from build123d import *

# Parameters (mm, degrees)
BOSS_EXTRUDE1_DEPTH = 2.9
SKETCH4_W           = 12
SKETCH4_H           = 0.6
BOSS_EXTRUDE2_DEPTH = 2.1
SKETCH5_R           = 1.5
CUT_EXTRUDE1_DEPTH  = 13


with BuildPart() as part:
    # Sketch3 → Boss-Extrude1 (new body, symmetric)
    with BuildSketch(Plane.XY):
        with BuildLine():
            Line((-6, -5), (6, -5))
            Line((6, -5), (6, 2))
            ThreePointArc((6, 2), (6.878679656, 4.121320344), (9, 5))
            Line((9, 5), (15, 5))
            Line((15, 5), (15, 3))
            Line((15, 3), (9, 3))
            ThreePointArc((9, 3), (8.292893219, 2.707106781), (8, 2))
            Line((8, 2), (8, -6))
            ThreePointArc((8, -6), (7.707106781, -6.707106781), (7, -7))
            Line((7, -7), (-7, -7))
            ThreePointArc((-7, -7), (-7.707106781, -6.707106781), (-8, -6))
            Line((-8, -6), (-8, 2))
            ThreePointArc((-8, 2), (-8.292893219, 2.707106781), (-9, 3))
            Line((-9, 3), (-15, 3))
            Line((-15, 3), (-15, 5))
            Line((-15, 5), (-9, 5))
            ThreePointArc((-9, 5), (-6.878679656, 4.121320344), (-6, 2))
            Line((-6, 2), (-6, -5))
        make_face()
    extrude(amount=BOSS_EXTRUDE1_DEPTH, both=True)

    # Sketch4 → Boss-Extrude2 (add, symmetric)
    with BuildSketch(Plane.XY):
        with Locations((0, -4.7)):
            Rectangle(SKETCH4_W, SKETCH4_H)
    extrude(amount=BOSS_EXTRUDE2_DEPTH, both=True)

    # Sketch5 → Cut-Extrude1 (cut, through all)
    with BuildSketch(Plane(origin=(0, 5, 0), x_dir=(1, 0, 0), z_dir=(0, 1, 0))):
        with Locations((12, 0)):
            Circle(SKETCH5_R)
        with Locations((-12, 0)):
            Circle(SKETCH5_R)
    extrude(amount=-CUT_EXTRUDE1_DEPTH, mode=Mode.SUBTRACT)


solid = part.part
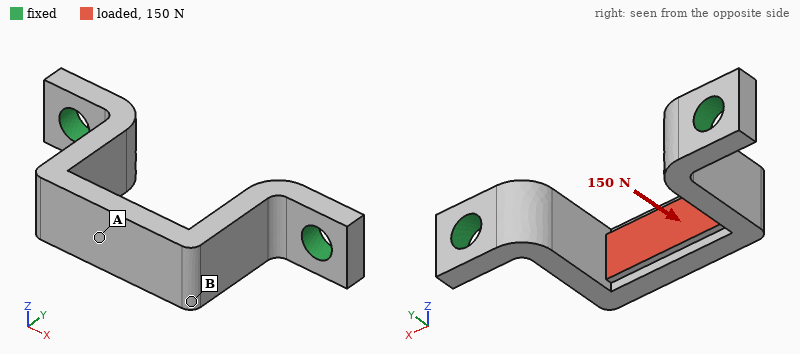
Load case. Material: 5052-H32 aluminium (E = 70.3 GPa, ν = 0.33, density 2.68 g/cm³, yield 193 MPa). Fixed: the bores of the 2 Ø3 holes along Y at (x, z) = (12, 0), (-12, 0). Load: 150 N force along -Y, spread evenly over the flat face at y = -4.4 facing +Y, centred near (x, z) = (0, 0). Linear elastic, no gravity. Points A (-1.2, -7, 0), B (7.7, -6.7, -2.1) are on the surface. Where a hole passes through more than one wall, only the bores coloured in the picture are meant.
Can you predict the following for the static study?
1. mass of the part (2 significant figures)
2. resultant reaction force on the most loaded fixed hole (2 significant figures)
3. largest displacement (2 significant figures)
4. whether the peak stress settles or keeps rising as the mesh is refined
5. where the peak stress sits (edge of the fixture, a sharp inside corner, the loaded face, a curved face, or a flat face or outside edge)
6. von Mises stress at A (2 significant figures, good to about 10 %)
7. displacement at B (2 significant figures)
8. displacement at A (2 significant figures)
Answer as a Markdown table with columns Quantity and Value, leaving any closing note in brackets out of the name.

| Quantity | Value |
|---|---|
| mass of the part | 1.5 g |
| resultant reaction force on the most loaded fixed hole | 81 N |
| largest displacement | 8.5 µm |
| whether the peak stress settles or keeps rising as the mesh is refined | keeps rising |
| where the peak stress sits | edge of the fixture |
| von Mises stress at A | 25 MPa |
| displacement at B | 2.9 µm |
| displacement at A | 8.0 µm |
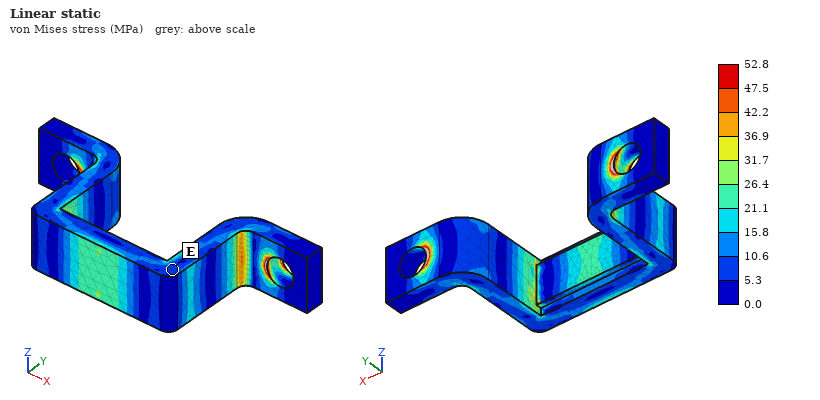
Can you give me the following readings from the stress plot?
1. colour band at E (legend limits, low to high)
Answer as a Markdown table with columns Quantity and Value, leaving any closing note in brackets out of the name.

| Quantity | Value |
|---|---|
| colour band at E | 5.3 to 10.6 MPa |
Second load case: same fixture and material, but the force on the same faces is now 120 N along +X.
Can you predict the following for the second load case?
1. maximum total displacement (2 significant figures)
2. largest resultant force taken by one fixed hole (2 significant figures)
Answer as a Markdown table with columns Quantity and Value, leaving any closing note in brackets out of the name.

| Quantity | Value |
|---|---|
| maximum total displacement | 28 µm |
| largest resultant force taken by one fixed hole | 70 N |
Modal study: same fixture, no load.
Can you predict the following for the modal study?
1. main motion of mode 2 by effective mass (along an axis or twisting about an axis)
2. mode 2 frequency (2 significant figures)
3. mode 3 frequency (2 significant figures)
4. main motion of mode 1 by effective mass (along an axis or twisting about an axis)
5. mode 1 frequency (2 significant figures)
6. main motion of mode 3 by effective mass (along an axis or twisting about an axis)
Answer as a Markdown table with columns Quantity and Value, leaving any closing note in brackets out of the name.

| Quantity | Value |
|---|---|
| main motion of mode 2 by effective mass | along X |
| mode 2 frequency | 12 kHz |
| mode 3 frequency | 17 kHz |
| main motion of mode 1 by effective mass | along Z |
| mode 1 frequency | 8500 Hz |
| main motion of mode 3 by effective mass | twisting about Y |
